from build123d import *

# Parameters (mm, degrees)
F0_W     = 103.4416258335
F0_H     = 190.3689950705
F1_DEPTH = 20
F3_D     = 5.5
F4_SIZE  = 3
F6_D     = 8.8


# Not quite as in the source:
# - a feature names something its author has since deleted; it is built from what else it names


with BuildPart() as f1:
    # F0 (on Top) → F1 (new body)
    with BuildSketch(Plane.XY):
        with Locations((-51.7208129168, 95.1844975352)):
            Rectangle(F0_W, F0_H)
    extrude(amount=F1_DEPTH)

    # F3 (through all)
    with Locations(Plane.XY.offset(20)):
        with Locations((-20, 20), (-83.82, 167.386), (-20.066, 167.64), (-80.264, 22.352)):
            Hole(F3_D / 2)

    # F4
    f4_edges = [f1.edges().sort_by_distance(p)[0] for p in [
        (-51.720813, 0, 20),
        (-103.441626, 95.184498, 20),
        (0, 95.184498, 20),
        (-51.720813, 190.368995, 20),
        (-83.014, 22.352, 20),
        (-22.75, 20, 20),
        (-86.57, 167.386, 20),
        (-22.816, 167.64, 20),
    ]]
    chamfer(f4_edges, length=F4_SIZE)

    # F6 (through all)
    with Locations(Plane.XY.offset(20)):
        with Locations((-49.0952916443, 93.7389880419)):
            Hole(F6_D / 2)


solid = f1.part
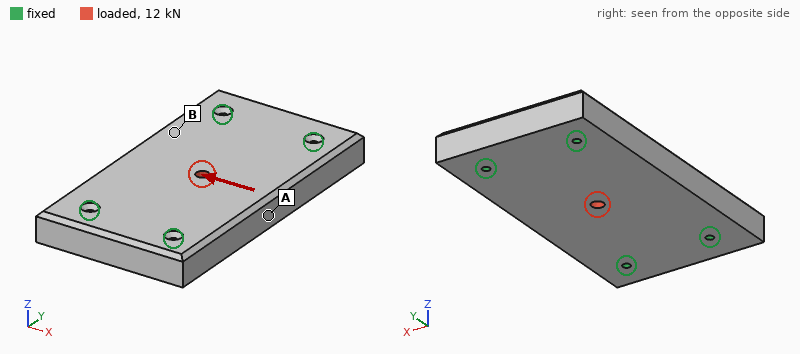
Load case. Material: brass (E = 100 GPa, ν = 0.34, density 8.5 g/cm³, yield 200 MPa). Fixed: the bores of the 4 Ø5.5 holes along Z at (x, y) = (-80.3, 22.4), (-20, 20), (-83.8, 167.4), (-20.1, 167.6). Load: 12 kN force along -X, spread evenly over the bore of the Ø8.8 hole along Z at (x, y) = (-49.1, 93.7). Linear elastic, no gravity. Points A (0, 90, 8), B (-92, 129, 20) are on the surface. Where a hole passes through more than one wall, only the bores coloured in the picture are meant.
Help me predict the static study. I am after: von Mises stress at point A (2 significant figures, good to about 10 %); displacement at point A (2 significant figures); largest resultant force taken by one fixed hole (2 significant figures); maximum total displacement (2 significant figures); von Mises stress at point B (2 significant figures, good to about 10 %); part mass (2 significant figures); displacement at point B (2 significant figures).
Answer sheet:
9.2 MPa
7.6 µm
4.2 kN
11 µm
3.6 MPa
3.3 kg
5.4 µm
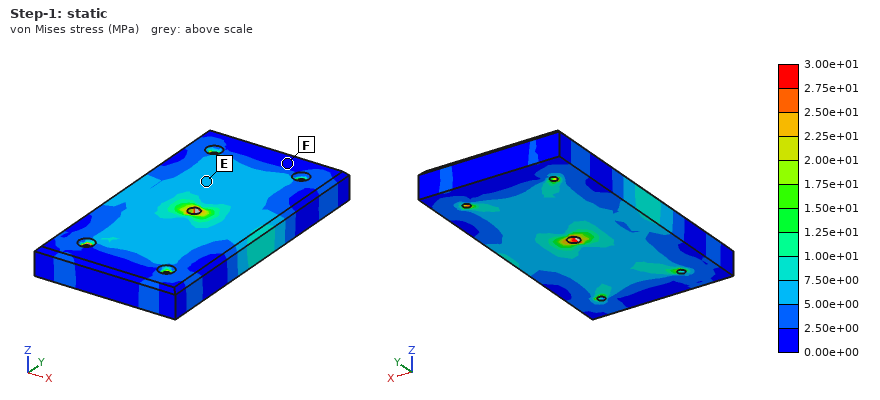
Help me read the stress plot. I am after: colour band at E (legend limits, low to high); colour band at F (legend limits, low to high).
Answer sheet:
5.00e+00 to 7.50e+00 MPa
0.00e+00 to 2.50e+00 MPa
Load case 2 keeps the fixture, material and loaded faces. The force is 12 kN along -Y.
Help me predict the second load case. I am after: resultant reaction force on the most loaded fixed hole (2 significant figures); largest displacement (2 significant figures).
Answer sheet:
3.1 kN
5.8 µm
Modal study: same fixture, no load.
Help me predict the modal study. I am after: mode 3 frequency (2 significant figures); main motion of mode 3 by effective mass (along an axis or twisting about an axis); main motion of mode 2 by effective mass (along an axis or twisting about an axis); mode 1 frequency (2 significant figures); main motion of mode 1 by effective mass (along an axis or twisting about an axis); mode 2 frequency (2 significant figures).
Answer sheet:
5400 Hz
along X
twisting about Y
2300 Hz
along Z
3400 Hz
